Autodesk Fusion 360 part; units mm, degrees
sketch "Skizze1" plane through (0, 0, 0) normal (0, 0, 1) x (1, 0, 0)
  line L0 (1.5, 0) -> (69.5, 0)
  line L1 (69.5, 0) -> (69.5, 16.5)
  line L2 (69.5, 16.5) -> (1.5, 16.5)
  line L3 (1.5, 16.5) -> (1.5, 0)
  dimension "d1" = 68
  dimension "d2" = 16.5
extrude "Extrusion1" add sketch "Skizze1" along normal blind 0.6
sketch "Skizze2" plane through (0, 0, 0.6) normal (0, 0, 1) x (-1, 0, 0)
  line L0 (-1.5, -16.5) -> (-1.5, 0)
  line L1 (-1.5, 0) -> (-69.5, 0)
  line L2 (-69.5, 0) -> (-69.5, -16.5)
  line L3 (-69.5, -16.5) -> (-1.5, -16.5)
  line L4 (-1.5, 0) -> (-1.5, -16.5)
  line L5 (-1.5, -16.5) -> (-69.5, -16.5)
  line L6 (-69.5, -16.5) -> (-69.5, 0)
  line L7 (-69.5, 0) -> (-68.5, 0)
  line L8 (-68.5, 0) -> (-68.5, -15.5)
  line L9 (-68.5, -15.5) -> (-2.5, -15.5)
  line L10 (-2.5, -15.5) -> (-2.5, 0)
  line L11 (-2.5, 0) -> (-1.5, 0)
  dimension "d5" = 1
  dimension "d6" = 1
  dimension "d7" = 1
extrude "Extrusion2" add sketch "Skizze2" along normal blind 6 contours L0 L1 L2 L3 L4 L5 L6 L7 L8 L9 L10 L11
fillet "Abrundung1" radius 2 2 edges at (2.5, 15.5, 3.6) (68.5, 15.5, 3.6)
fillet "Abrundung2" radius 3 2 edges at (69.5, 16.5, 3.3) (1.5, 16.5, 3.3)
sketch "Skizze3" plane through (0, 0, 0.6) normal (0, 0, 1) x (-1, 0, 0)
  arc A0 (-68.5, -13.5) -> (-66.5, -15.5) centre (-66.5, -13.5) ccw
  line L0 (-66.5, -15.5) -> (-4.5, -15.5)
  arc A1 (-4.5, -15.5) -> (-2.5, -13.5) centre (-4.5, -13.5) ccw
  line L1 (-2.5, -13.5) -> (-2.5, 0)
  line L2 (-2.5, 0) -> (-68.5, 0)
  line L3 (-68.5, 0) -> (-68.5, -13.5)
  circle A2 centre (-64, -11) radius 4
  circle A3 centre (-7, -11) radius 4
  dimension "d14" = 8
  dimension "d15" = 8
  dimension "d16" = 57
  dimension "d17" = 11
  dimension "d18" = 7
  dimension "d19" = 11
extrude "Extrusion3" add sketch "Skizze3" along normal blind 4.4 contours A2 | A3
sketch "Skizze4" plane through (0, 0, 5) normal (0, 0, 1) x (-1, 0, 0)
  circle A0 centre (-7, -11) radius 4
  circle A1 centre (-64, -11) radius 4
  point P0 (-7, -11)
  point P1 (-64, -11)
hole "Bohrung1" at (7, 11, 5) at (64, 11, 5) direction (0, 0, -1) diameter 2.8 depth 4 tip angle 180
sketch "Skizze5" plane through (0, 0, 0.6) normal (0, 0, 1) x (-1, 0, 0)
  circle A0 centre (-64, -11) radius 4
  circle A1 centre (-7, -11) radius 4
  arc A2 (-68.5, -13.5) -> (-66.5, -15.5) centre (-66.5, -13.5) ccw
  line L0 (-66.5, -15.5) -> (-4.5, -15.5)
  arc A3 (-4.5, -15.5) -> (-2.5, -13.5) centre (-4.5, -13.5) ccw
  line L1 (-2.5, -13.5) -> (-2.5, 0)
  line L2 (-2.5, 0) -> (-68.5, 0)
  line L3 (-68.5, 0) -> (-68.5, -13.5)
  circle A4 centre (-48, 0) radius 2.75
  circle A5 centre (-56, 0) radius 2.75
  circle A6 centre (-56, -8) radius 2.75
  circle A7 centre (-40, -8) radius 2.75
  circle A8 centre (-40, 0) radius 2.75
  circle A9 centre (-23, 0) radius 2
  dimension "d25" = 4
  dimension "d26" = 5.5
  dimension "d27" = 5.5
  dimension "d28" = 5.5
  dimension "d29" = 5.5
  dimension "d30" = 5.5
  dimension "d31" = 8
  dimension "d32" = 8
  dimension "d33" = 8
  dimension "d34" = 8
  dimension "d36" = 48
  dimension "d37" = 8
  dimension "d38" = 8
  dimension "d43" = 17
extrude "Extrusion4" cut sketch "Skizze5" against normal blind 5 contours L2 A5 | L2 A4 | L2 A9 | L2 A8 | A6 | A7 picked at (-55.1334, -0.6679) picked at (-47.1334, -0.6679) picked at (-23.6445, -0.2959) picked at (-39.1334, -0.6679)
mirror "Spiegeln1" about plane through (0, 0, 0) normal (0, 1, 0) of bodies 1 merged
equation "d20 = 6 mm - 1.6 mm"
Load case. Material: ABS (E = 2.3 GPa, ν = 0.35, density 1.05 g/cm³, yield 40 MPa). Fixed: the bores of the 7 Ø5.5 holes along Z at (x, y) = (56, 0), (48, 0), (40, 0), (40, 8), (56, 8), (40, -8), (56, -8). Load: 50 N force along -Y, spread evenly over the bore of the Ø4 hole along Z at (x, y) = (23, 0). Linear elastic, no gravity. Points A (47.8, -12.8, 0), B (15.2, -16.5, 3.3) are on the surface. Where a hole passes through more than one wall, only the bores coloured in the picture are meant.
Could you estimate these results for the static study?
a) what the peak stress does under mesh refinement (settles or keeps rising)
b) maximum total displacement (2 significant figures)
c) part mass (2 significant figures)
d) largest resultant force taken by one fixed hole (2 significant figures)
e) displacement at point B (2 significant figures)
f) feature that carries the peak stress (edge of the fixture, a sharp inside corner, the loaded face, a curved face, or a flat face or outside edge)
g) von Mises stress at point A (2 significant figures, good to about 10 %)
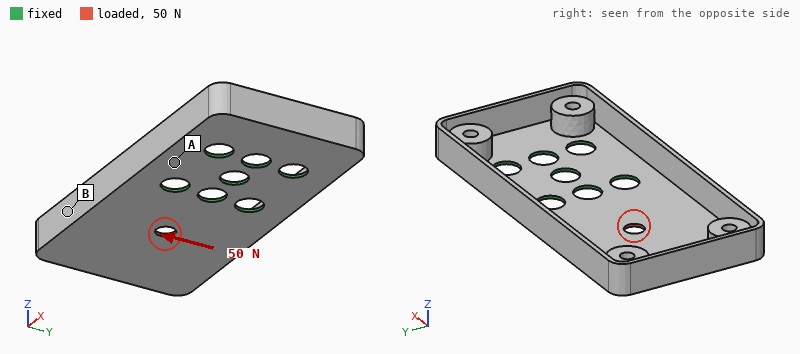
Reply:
keeps rising
0.22 mm
3.3 g
33 N
0.15 mm
edge of the fixture
1.8 MPa
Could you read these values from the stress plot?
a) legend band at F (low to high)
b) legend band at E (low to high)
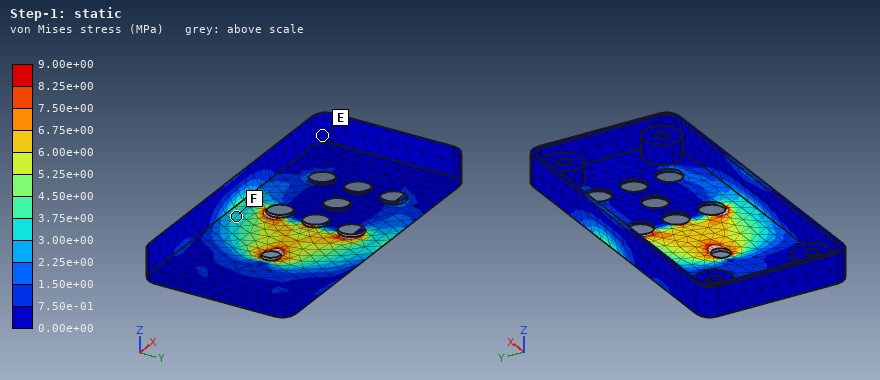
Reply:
3.00e+00 to 3.75e+00 MPa
0.00e+00 to 7.50e-01 MPa
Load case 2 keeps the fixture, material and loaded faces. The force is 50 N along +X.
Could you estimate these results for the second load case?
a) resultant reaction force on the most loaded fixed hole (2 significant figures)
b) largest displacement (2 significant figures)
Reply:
17 N
73 µm
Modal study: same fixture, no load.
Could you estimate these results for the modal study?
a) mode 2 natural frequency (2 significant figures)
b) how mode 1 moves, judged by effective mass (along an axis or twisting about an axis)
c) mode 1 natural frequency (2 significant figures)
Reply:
350 Hz
along Z
280 Hz
